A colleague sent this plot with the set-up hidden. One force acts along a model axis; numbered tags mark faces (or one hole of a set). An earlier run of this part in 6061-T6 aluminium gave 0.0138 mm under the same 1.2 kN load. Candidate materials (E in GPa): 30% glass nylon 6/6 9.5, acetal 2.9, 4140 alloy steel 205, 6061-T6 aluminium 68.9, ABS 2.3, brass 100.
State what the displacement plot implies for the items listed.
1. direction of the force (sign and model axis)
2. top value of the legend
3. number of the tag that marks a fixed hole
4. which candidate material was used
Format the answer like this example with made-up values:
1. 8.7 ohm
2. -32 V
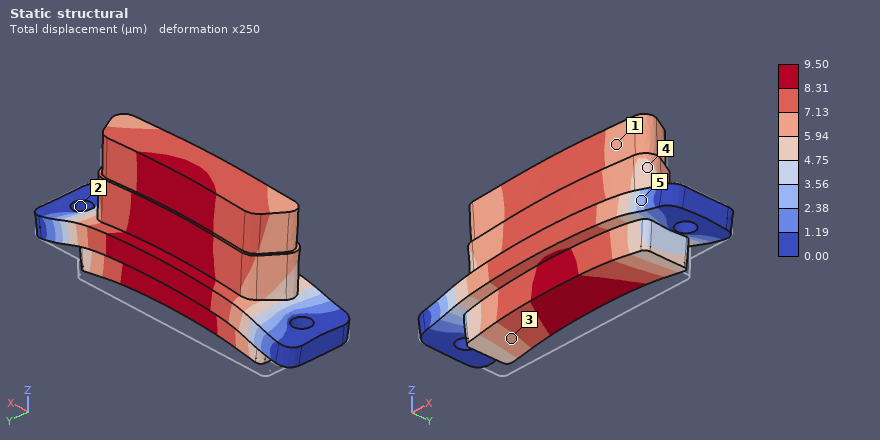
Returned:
1. +Z
2. 9.50 µm
3. 2
4. brass
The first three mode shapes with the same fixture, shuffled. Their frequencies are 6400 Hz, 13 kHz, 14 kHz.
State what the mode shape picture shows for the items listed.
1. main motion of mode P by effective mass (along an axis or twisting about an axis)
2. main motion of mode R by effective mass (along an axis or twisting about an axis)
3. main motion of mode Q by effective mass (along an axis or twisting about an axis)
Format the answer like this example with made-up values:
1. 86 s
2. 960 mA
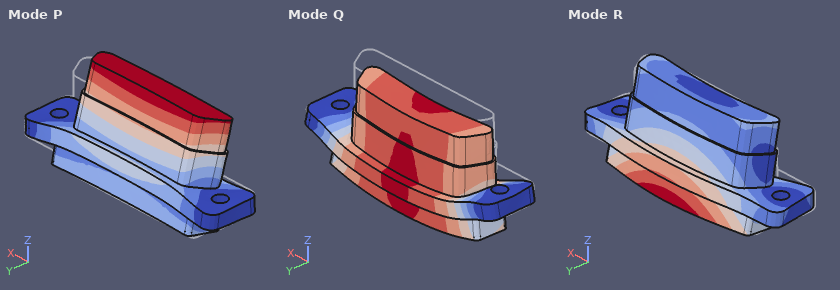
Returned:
1. along Y
2. along Y
3. along Z
